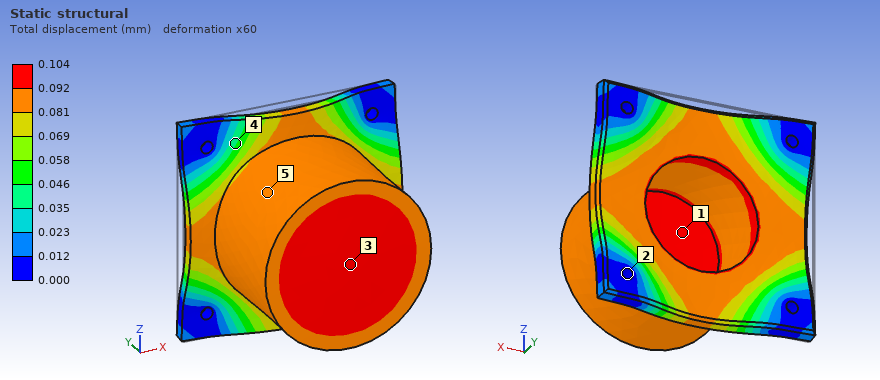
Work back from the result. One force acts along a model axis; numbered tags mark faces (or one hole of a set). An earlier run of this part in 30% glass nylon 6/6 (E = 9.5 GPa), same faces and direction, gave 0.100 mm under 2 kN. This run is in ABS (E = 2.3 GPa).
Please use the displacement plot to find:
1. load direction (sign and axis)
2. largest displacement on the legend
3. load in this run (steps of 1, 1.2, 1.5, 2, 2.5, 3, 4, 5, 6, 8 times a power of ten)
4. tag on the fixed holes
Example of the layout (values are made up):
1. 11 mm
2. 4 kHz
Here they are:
1. -Y
2. 0.104 mm
3. 500 N
4. 2
